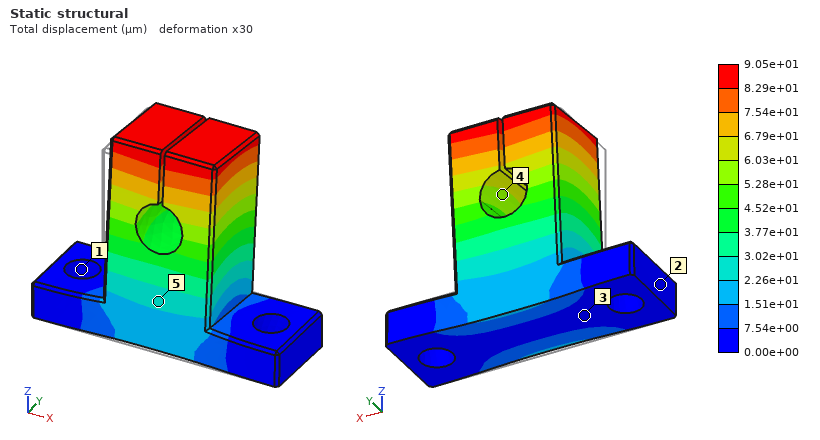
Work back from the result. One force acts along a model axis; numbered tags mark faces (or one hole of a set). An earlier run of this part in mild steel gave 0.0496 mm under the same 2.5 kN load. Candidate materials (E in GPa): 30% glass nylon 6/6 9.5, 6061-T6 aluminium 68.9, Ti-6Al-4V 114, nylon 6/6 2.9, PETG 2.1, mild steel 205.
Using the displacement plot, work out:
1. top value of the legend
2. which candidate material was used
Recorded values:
9.05e+01 µm
Ti-6Al-4V
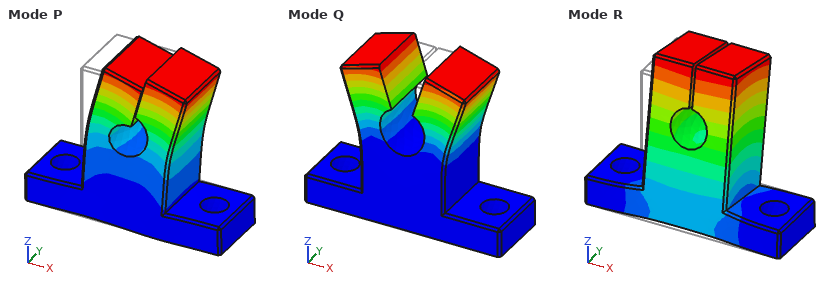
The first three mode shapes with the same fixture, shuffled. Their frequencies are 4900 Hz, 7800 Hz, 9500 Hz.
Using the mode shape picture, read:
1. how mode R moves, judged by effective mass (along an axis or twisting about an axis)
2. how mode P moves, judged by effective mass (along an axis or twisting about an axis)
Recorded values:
along Y
along X
